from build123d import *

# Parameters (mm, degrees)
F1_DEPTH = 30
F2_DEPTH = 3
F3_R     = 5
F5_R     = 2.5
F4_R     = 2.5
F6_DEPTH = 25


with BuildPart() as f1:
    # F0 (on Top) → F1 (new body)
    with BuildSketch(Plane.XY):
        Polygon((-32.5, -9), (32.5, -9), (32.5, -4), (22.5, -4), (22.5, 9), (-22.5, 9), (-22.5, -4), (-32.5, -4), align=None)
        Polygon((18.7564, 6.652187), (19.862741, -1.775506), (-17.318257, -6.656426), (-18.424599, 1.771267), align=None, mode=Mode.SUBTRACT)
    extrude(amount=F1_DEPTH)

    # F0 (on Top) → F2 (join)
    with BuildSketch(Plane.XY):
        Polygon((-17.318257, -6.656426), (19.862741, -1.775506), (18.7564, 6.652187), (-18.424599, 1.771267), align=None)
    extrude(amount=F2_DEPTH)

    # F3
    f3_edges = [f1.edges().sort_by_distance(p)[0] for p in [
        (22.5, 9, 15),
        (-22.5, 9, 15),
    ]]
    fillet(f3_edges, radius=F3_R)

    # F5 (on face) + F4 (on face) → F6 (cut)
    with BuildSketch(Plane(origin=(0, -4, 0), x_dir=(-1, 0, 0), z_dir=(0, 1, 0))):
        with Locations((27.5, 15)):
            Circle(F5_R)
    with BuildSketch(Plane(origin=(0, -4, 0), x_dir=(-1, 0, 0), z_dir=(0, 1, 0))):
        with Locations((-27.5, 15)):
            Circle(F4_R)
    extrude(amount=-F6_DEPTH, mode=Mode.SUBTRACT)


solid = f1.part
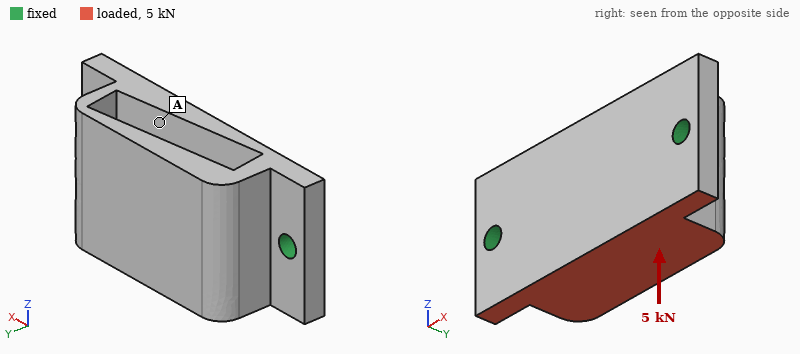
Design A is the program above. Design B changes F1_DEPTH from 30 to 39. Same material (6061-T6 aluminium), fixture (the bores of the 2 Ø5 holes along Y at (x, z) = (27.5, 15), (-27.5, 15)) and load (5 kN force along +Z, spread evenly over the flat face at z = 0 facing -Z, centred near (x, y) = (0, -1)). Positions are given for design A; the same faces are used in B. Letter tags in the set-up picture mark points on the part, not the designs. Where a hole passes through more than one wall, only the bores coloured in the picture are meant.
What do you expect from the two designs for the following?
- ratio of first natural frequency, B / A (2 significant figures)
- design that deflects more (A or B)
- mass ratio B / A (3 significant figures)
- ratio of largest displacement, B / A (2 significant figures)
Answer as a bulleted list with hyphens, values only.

- 0.73
- B
- 1.29
- 1.2
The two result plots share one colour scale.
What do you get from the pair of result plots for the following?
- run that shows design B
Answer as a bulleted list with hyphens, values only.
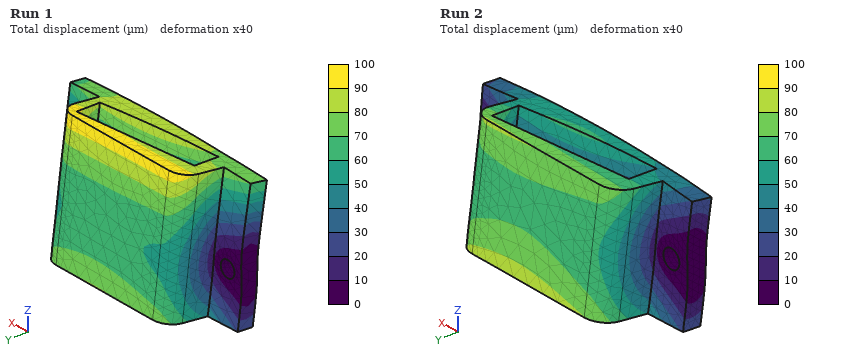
- Run 1
